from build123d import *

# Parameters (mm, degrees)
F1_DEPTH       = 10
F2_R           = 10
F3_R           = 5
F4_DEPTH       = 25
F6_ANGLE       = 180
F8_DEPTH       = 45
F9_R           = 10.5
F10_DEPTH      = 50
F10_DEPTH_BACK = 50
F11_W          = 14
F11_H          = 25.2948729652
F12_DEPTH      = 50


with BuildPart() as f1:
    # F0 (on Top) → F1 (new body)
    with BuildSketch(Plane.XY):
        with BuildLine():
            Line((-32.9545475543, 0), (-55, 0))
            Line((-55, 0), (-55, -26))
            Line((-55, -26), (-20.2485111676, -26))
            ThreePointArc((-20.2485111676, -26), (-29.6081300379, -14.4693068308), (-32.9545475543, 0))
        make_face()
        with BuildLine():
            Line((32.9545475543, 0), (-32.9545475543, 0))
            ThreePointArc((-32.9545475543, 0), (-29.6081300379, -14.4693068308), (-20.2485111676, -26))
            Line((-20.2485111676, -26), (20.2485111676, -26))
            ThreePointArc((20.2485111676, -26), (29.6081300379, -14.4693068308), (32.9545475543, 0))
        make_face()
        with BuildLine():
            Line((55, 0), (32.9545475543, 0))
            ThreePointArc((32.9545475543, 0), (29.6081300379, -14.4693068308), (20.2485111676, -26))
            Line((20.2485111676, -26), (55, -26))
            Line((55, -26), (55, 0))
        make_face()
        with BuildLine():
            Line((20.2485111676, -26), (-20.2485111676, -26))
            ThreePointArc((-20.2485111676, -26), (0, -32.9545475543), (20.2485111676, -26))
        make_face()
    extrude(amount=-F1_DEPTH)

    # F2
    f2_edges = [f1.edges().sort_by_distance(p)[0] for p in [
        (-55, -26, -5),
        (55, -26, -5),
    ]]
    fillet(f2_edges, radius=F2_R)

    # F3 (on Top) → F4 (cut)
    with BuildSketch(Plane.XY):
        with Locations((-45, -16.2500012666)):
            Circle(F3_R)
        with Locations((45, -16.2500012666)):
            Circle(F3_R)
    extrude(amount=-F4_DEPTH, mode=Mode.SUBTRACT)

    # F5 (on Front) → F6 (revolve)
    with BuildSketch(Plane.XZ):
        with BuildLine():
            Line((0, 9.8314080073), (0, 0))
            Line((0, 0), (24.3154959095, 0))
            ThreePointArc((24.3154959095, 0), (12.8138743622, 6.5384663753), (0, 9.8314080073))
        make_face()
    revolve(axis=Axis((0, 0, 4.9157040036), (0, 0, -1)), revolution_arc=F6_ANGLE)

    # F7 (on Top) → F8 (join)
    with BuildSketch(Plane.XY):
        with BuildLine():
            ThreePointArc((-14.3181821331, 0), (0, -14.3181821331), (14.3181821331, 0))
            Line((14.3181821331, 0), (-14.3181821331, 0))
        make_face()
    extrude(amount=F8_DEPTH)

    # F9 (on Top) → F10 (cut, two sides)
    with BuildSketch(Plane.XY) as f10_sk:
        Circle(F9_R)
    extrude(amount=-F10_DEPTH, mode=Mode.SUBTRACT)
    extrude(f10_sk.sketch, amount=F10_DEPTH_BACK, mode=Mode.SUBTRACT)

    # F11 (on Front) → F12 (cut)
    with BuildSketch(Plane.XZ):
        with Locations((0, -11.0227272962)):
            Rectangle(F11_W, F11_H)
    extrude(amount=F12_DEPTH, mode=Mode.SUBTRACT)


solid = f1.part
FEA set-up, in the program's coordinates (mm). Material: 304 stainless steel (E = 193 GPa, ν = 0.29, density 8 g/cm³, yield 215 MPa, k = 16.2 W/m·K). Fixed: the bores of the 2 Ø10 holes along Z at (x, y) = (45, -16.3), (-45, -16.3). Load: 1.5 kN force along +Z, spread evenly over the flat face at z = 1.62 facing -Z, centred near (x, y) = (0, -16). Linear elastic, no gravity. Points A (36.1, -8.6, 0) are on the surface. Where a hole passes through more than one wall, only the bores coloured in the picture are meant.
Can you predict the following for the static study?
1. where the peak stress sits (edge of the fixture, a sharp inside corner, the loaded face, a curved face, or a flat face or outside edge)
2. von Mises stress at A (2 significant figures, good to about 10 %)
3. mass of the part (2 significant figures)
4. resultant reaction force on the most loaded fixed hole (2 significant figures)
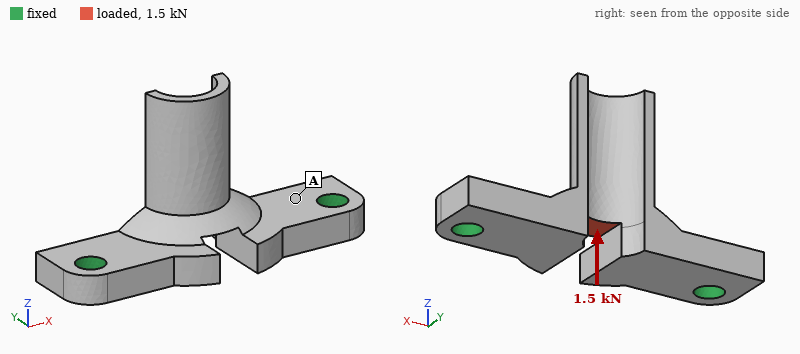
a curved face
13 MPa
250 g
1.5 kN
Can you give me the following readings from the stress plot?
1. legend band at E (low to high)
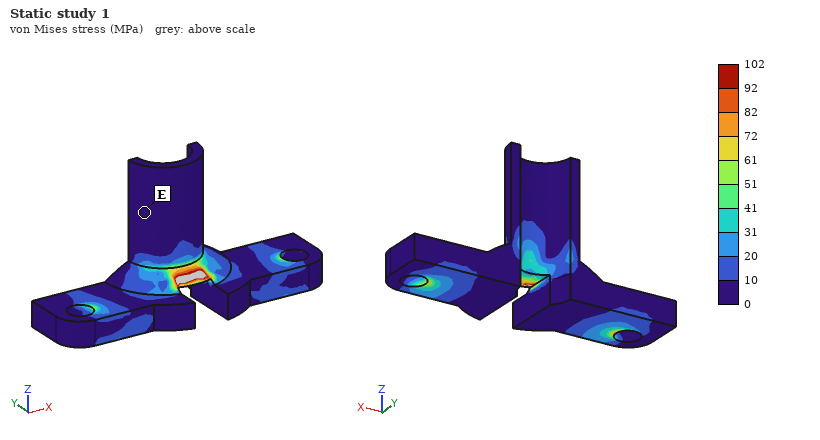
0 to 10 MPa
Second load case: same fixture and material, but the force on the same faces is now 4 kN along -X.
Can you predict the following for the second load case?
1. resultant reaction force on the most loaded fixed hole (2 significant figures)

2.0 kN
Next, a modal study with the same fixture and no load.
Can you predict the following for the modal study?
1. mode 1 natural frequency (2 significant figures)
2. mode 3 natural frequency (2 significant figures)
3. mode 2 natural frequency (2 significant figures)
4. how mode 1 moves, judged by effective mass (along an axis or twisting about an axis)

3000 Hz
5200 Hz
3900 Hz
along Y
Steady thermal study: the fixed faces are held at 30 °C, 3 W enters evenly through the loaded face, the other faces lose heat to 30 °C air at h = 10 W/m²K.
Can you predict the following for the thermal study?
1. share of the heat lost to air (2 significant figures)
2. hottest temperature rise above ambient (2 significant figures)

25 %
32 K
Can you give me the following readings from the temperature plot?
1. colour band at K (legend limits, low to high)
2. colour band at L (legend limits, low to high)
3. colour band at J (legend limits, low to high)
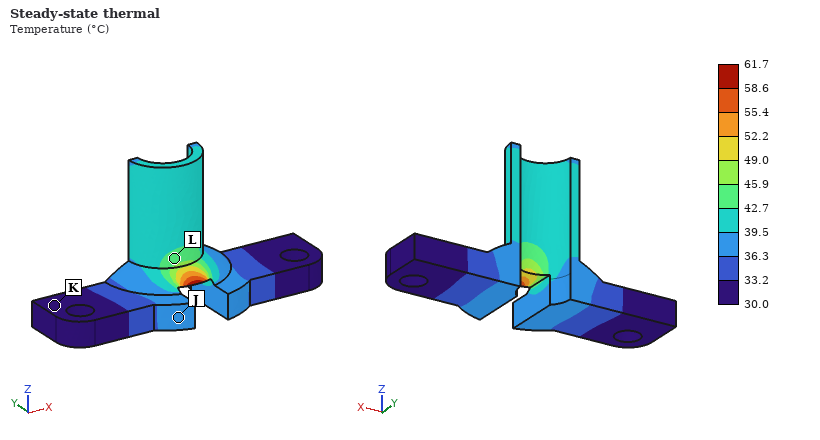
30.0 to 33.2 °C
42.7 to 45.9 °C
36.3 to 39.5 °C
